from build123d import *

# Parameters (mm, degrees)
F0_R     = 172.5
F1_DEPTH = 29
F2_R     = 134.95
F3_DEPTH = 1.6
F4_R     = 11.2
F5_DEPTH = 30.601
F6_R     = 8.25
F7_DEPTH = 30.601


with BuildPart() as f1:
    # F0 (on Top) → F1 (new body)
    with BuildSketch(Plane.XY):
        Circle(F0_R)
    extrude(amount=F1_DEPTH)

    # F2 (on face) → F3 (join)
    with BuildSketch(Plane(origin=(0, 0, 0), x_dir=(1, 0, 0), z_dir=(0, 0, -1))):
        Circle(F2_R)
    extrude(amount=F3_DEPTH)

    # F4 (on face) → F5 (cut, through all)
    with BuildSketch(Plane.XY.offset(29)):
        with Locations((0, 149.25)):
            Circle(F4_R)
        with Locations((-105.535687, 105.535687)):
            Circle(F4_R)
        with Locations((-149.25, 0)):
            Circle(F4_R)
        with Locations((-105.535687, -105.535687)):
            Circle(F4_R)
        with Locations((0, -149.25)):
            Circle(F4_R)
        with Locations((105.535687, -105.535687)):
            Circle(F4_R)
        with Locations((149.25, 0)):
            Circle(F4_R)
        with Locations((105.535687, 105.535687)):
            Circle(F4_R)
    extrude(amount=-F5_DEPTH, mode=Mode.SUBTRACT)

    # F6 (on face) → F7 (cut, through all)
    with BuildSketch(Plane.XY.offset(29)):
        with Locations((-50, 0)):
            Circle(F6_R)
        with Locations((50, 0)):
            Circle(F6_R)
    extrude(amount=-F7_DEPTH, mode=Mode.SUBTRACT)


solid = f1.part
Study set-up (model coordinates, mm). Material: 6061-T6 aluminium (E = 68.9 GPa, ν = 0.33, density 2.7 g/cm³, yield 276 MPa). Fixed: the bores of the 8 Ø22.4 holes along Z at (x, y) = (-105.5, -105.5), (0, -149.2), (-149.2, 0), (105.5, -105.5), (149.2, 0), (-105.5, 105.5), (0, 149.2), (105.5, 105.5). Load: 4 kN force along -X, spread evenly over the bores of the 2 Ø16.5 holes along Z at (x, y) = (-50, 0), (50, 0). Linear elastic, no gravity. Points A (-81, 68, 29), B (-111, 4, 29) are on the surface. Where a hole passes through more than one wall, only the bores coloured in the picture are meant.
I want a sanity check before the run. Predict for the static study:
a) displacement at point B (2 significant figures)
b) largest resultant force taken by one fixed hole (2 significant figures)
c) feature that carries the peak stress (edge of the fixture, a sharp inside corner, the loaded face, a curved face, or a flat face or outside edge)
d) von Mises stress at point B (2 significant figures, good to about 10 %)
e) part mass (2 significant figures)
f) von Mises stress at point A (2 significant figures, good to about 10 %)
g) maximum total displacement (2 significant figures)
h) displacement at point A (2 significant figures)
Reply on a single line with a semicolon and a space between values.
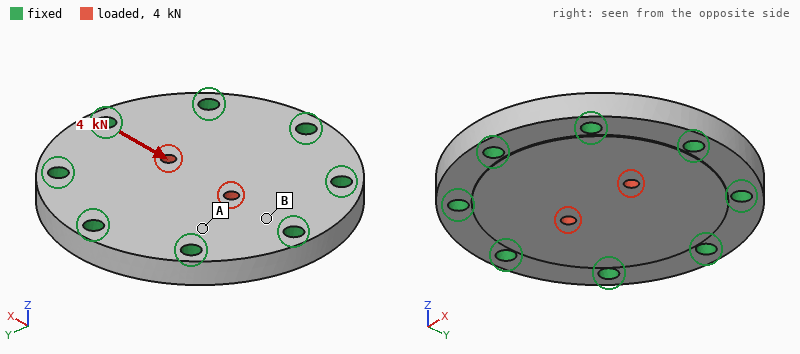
0.28 µm; 960 N; the loaded face; 0.63 MPa; 7.3 kg; 0.28 MPa; 1.0 µm; 0.22 µm
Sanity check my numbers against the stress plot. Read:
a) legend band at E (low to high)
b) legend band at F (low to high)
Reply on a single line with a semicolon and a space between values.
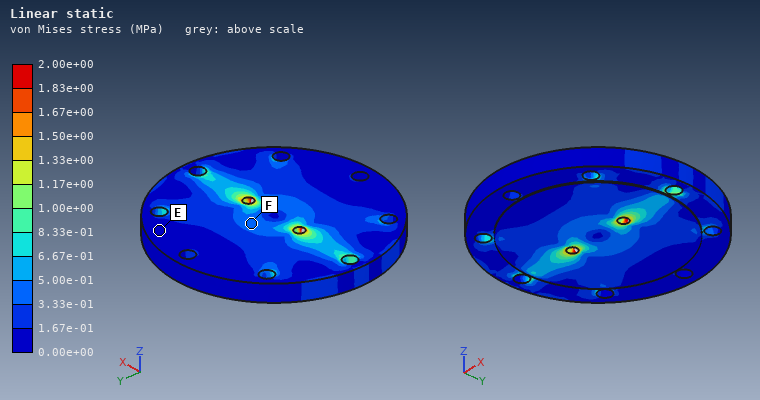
0.00e+00 to 1.67e-01 MPa; 3.33e-01 to 5.00e-01 MPa
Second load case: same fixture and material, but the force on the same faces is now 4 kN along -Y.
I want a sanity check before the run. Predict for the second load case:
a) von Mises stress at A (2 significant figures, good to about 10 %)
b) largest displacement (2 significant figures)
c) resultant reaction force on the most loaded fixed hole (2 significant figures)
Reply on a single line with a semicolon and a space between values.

0.38 MPa; 0.87 µm; 690 N
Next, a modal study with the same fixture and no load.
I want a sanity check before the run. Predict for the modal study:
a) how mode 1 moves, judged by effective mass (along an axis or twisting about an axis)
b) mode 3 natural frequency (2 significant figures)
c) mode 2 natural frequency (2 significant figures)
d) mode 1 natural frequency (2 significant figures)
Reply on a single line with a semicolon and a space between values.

along Z; 5500 Hz; 5500 Hz; 2800 Hz
